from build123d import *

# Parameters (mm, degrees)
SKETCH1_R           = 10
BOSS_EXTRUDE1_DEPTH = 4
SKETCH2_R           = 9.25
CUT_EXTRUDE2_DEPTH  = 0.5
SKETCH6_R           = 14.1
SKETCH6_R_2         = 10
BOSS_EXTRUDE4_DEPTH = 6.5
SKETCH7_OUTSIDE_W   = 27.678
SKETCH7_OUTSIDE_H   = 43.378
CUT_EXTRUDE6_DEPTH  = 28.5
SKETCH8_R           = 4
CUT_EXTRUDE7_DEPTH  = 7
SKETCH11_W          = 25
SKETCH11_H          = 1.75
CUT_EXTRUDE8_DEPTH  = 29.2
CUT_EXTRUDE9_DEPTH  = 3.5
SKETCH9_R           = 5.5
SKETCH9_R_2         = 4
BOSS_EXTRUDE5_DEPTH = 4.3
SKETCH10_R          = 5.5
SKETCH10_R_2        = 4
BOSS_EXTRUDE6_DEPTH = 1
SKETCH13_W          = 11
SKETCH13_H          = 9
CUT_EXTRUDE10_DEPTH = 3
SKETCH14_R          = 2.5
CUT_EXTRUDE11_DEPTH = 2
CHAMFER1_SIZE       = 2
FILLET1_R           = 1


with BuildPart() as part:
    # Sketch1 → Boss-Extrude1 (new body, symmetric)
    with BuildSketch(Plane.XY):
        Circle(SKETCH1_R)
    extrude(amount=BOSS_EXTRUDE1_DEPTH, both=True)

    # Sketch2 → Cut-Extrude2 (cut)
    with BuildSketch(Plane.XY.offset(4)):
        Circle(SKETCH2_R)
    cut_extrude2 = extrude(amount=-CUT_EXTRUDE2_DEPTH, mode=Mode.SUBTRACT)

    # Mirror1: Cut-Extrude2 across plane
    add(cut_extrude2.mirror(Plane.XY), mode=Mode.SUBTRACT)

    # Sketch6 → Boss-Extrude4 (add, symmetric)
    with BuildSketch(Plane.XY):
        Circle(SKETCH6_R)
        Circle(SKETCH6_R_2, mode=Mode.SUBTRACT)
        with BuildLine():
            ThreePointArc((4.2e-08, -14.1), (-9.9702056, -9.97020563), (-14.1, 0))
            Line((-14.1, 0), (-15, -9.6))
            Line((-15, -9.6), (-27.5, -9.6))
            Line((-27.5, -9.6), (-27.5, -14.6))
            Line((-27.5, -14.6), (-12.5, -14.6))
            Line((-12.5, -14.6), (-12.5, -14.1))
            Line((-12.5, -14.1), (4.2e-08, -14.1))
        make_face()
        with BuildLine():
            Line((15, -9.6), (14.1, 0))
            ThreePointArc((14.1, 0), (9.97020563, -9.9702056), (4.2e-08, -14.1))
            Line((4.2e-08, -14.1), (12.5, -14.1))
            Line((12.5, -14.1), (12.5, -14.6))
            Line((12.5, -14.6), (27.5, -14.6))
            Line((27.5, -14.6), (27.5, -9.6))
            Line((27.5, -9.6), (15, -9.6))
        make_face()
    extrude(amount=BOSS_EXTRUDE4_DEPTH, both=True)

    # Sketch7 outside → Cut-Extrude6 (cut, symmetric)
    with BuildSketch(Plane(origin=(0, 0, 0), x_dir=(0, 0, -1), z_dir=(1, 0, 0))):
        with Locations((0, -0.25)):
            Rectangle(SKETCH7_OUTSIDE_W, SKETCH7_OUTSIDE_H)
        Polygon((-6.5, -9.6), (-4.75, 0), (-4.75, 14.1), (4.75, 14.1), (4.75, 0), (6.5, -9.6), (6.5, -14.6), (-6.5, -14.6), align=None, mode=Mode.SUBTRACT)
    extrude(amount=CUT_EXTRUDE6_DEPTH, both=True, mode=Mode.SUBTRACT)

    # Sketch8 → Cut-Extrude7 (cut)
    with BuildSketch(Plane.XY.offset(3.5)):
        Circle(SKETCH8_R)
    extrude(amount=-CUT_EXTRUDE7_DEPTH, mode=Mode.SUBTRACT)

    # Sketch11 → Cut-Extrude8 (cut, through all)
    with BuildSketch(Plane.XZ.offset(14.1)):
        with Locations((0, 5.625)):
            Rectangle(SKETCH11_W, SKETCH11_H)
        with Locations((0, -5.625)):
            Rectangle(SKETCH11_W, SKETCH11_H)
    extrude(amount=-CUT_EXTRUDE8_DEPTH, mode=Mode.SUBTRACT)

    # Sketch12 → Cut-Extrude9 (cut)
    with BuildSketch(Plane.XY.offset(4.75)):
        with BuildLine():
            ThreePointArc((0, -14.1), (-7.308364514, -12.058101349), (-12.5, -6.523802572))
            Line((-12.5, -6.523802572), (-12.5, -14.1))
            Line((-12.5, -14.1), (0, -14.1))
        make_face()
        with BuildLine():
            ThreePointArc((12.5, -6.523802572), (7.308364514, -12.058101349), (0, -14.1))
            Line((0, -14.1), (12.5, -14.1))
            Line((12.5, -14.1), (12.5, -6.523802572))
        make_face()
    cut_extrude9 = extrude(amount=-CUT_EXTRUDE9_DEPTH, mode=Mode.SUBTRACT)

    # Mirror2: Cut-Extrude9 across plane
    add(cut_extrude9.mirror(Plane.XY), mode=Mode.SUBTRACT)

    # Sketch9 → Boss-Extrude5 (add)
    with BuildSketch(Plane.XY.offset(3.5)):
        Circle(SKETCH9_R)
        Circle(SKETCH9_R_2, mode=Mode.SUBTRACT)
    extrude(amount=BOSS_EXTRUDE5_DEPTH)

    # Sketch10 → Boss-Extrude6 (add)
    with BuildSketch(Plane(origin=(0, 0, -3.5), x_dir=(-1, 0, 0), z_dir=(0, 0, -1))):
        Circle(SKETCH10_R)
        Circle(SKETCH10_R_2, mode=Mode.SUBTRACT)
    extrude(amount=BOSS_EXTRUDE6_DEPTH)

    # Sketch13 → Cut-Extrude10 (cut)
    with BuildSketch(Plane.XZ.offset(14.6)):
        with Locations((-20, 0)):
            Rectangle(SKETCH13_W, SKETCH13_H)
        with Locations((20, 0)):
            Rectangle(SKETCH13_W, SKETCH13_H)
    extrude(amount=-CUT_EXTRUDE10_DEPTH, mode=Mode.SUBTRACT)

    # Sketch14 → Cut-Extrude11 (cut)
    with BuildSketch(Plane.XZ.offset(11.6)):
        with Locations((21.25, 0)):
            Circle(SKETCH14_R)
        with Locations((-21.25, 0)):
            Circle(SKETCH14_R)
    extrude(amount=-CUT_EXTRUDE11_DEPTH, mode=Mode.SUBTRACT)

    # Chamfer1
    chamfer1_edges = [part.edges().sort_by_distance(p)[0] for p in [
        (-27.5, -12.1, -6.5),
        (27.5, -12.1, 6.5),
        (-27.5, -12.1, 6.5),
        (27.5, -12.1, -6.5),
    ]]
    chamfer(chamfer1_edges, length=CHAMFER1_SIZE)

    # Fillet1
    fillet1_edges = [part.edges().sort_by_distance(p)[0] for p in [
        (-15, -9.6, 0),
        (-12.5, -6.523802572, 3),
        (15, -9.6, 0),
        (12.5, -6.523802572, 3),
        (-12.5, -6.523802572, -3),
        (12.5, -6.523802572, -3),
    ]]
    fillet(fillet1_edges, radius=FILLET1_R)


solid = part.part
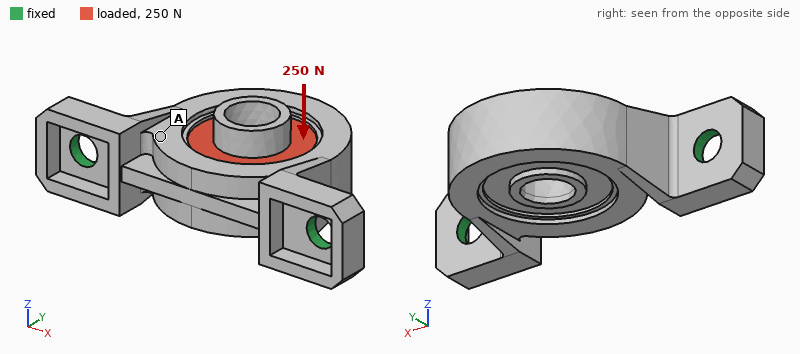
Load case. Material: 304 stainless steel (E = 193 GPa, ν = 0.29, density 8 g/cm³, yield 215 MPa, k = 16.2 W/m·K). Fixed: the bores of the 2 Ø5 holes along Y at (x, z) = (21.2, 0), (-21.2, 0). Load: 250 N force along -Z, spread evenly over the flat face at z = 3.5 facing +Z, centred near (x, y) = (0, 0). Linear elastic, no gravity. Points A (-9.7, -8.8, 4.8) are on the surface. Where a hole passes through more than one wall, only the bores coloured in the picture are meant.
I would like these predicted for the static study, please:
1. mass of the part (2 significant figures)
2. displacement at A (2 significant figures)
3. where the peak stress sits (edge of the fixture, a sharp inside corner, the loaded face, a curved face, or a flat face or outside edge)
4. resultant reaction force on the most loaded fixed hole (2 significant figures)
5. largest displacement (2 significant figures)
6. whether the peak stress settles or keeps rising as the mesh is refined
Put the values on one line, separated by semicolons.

54 g; 5.5 µm; edge of the fixture; 130 N; 26 µm; keeps rising
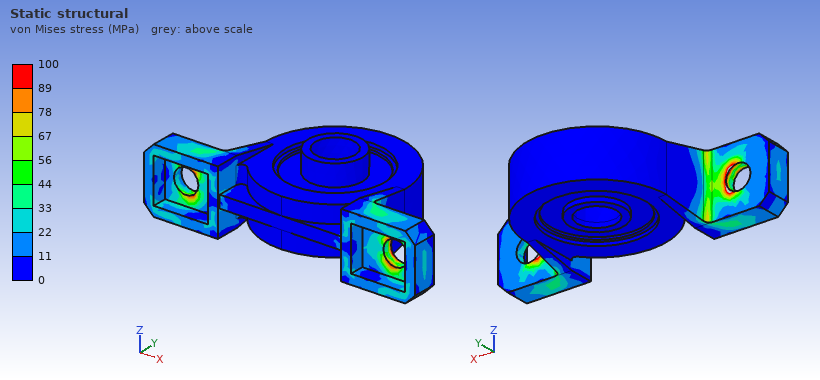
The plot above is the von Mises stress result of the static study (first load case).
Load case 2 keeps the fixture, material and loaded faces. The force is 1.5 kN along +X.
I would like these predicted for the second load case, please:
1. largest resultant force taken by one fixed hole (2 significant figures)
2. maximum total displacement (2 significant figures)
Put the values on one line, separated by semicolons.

890 N; 10.0 µm
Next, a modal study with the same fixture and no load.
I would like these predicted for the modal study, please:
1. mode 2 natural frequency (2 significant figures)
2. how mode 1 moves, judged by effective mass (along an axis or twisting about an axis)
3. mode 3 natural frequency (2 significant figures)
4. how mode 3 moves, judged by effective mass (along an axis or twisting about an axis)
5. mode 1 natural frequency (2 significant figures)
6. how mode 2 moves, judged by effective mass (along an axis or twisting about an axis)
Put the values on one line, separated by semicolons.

9400 Hz; along Z; 11 kHz; along X; 3000 Hz; along Y
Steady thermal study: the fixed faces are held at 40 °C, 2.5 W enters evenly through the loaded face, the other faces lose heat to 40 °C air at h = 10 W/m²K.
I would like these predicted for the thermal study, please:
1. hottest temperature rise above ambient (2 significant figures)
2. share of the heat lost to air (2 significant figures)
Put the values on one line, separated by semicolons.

24 K; 24 %
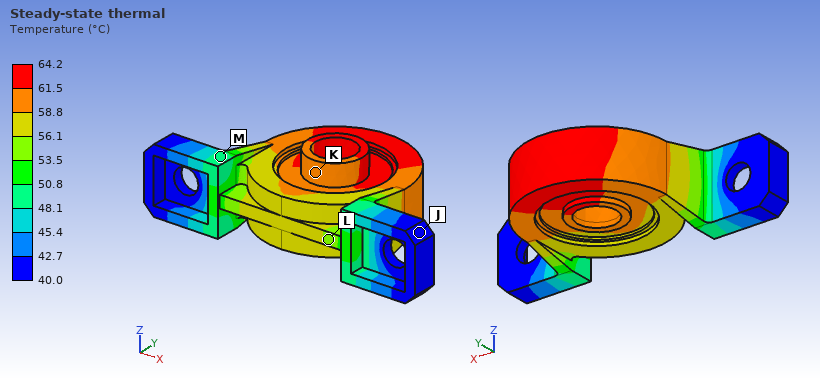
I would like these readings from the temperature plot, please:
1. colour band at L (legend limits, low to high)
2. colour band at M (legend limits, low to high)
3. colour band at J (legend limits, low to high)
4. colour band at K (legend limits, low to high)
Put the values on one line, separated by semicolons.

53.5 to 56.1 °C; 48.1 to 50.8 °C; 40.0 to 42.7 °C; 58.8 to 61.5 °C
